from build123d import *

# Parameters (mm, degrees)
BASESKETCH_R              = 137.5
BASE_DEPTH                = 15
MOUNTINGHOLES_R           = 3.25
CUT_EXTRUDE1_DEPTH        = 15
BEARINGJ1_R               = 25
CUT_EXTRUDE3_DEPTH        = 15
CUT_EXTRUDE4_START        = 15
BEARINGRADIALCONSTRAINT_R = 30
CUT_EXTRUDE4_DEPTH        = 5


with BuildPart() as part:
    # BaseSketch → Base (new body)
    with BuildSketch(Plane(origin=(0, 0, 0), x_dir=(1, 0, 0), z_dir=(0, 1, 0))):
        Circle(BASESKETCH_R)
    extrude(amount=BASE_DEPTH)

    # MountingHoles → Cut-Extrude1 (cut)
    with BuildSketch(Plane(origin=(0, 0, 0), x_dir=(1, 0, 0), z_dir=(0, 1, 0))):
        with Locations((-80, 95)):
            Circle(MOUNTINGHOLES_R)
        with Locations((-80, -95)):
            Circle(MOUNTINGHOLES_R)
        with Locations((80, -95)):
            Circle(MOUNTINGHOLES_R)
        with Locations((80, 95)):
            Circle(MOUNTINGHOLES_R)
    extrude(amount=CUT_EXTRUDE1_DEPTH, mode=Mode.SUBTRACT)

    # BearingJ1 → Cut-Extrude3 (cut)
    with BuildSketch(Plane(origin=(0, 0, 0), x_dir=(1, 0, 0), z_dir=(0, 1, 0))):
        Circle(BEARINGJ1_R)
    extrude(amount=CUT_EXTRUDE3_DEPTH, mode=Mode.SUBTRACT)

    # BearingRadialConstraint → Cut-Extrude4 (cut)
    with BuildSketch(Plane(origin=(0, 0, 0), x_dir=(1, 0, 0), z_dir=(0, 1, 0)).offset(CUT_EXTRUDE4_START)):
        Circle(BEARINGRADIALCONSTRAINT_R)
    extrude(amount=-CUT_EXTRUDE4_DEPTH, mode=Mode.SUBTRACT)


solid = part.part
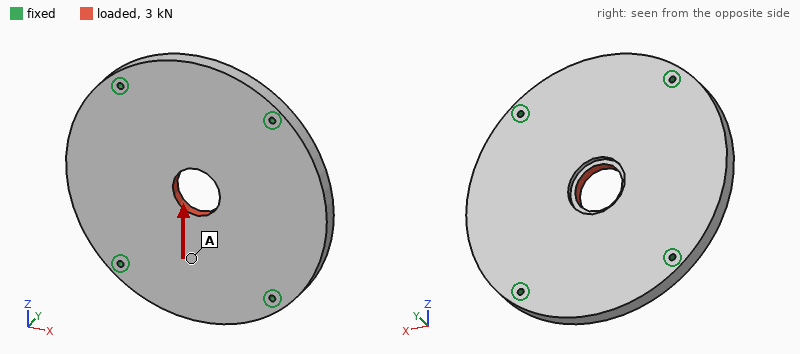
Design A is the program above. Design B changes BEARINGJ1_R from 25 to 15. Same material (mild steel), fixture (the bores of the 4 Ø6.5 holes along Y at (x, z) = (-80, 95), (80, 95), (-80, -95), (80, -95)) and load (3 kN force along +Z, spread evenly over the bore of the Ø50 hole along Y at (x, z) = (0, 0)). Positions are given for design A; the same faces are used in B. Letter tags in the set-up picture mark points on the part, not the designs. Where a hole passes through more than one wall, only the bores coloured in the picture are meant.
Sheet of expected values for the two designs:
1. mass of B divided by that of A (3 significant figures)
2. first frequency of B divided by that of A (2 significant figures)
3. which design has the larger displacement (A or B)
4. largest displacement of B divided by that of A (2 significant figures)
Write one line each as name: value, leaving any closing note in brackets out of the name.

mass of B divided by that of A: 1.01
first frequency of B divided by that of A: 0.99
which design has the larger displacement: B
largest displacement of B divided by that of A: 1.2
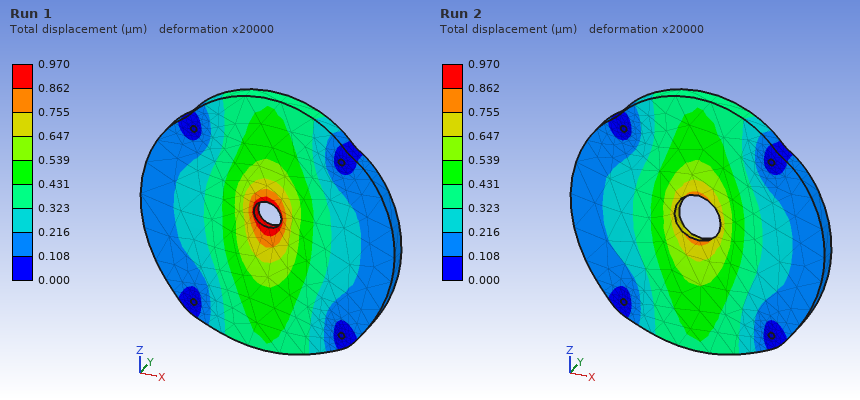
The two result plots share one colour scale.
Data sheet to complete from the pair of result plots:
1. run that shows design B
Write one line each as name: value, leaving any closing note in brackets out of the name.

run that shows design B: Run 1
